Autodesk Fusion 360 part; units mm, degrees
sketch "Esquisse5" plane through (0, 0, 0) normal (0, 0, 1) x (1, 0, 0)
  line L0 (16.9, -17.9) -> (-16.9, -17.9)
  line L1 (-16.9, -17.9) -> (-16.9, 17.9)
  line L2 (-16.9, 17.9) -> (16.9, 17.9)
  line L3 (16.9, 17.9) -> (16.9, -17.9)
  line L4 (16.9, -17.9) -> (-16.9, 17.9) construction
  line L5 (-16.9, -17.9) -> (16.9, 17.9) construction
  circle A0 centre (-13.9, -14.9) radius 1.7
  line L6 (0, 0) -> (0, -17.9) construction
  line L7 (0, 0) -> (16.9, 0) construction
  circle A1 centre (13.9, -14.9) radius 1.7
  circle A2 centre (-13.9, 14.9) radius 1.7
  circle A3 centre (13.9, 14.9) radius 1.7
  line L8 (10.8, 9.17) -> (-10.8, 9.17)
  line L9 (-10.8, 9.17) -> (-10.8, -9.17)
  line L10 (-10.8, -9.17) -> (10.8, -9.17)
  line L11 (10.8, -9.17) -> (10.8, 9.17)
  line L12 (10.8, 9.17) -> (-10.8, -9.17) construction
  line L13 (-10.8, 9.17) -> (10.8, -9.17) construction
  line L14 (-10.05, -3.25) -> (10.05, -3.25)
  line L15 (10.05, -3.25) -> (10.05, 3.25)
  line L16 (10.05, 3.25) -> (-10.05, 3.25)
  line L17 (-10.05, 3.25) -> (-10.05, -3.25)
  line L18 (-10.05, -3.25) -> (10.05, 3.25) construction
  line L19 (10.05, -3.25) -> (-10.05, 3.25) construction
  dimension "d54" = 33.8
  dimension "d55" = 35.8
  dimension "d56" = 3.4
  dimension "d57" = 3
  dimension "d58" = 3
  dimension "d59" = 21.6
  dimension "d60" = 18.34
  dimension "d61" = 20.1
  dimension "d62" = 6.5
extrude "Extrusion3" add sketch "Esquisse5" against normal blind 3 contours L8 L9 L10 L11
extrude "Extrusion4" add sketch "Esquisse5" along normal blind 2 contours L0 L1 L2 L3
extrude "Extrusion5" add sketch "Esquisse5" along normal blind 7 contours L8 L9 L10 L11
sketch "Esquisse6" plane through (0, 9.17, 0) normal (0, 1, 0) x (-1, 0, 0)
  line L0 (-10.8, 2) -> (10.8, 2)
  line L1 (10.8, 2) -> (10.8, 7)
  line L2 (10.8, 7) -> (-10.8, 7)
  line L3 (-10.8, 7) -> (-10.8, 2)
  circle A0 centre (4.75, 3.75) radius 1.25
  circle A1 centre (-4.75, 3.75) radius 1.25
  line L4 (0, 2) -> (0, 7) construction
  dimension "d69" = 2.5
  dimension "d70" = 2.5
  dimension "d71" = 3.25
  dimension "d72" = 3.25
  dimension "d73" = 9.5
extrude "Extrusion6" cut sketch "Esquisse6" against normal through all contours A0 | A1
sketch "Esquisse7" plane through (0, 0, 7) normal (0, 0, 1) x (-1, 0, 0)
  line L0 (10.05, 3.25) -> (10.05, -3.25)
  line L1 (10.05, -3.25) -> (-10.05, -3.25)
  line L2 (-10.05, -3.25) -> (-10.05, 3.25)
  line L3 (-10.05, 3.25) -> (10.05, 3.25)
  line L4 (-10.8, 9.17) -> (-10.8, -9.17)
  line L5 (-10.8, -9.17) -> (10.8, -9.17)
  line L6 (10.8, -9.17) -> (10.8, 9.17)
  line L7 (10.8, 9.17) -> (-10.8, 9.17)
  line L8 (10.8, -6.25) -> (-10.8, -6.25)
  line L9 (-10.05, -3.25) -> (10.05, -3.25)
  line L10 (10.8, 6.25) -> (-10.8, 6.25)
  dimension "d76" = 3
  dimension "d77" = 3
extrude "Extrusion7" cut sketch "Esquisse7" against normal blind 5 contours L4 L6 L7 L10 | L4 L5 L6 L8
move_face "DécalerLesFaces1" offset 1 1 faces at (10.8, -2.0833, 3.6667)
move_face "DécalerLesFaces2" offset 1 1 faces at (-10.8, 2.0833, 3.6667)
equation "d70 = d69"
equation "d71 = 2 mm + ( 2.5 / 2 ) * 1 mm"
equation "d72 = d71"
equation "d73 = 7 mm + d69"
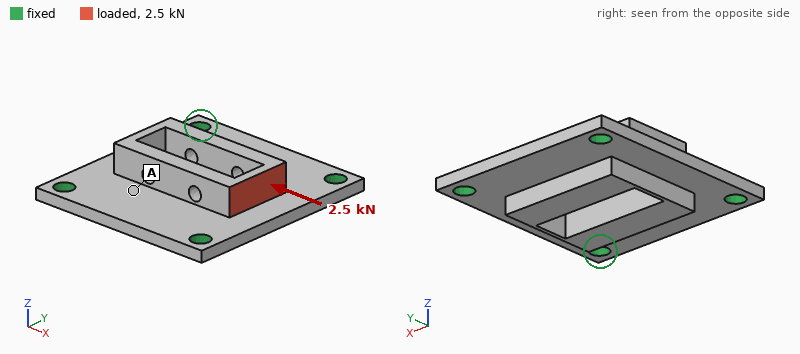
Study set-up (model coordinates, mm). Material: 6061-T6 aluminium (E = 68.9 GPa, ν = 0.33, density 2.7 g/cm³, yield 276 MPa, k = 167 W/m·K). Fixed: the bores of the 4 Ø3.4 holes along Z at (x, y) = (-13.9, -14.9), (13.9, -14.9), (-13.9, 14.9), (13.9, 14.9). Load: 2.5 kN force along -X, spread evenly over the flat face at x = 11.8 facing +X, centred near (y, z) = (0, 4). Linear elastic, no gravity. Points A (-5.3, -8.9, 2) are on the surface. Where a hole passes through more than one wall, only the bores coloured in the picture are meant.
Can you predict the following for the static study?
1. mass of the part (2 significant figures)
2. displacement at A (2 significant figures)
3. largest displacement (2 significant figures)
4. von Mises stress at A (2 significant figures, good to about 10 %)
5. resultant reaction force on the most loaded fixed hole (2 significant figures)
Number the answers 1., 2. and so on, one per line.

1. 9.8 g
2. 12 µm
3. 70 µm
4. 61 MPa
5. 750 N
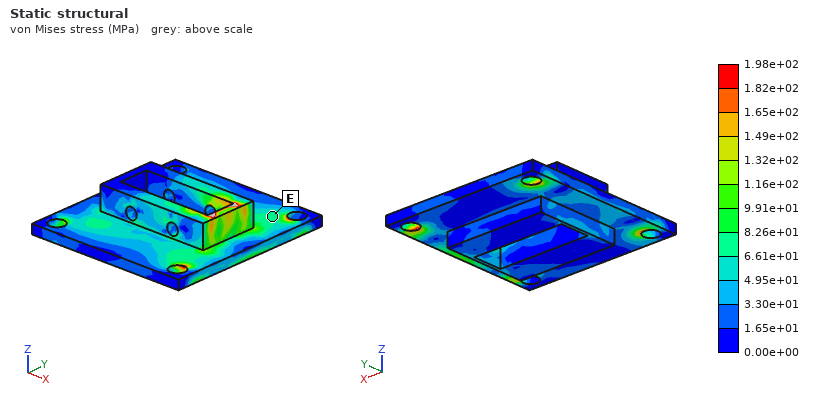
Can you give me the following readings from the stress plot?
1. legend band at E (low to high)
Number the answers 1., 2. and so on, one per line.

1. 6.61e+01 to 8.26e+01 MPa
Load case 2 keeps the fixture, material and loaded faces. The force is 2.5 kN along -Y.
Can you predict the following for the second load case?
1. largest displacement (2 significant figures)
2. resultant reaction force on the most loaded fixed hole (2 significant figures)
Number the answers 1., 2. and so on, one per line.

1. 56 µm
2. 1.2 kN
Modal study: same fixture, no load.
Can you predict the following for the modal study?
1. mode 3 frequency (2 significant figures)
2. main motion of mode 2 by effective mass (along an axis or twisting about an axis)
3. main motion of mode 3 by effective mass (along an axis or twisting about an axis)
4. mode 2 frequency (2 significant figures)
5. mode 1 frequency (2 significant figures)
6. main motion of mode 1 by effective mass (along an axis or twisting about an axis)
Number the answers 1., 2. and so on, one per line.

1. 17 kHz
2. twisting about Y
3. twisting about X
4. 15 kHz
5. 10 kHz
6. along Z
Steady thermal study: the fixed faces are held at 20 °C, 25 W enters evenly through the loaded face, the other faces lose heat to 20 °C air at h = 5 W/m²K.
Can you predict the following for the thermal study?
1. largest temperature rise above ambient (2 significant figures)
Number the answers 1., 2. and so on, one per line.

1. 38 K
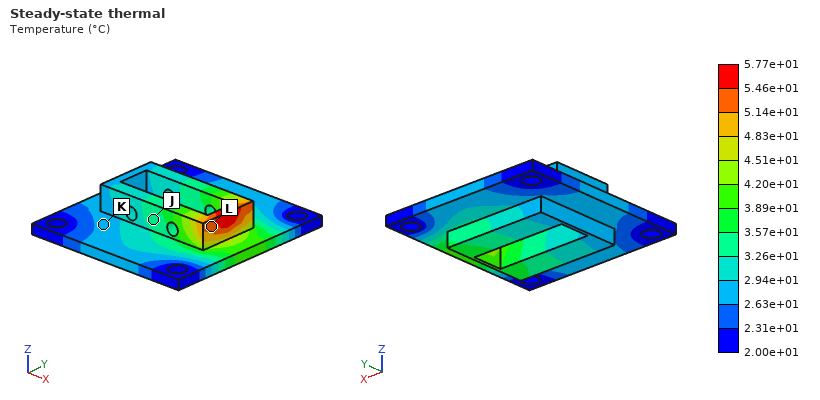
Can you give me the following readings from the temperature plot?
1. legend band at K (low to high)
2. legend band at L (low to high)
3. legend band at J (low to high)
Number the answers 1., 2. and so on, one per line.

1. 2.63e+01 to 2.94e+01 °C
2. 5.14e+01 to 5.46e+01 °C
3. 3.26e+01 to 3.57e+01 °C
